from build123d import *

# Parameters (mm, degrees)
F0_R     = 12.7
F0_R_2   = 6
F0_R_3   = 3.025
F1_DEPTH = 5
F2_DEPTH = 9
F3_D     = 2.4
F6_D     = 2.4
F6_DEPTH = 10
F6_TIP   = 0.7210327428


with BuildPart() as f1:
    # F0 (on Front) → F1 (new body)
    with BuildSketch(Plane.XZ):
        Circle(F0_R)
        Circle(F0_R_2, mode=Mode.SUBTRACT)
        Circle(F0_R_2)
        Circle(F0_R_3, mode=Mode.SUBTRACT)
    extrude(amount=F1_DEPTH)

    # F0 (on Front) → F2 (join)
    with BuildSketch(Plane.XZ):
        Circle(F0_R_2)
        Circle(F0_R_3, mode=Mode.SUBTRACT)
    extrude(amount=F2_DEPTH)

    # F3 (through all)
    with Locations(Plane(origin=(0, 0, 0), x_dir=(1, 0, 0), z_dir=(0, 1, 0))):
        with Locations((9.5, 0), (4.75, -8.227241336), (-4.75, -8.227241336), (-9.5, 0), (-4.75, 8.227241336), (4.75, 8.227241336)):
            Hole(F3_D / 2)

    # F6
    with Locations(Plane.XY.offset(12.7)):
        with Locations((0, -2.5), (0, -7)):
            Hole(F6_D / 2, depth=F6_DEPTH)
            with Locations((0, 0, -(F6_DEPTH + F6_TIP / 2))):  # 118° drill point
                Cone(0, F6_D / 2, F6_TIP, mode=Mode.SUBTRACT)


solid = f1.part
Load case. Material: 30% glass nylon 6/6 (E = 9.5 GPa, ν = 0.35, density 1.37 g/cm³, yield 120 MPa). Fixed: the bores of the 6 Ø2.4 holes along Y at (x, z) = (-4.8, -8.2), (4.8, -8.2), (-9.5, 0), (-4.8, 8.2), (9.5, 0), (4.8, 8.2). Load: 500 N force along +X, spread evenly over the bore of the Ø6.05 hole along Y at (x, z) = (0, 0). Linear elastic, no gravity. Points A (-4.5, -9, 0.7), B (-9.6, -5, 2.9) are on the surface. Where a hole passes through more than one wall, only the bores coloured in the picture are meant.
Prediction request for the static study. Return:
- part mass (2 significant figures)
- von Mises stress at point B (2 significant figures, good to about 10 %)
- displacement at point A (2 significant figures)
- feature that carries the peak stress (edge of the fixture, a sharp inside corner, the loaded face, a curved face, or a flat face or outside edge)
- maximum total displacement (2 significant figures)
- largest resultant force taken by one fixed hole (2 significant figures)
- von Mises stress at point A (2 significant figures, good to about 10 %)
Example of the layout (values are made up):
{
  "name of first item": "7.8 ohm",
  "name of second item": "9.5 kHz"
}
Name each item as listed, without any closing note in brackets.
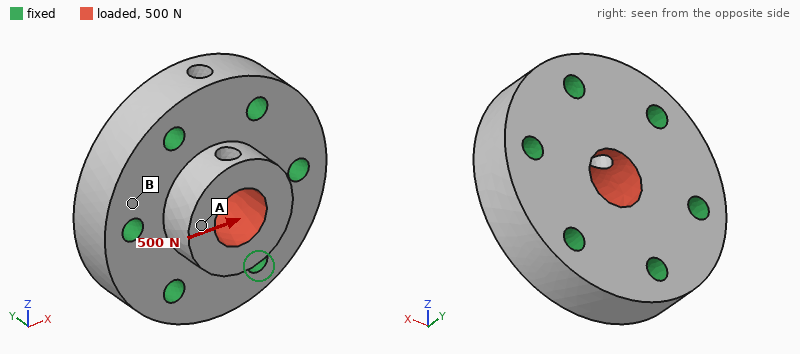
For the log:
{
  "part mass": "3.5 g",
  "von Mises stress at point B": "1.8 MPa",
  "displacement at point A": "7.9 µm",
  "feature that carries the peak stress": "the loaded face",
  "maximum total displacement": "8.6 µm",
  "largest resultant force taken by one fixed hole": "140 N",
  "von Mises stress at point A": "4.9 MPa"
}
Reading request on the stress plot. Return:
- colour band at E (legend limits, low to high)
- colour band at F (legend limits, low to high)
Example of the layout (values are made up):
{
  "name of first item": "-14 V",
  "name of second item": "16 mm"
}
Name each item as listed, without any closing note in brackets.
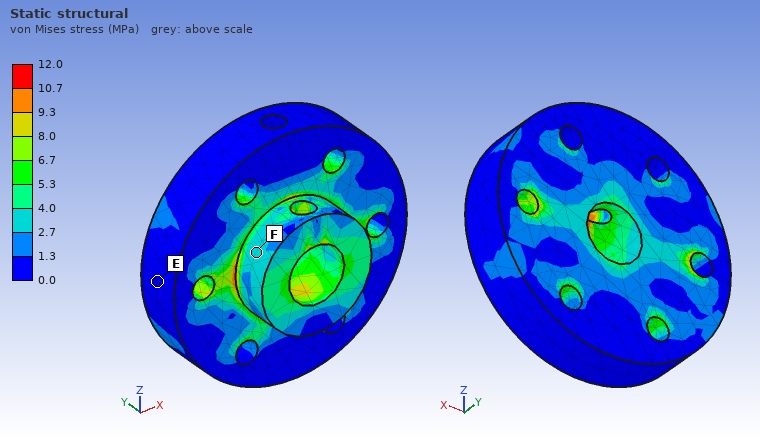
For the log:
{
  "colour band at E": "0.0 to 1.3 MPa",
  "colour band at F": "2.7 to 4.0 MPa"
}
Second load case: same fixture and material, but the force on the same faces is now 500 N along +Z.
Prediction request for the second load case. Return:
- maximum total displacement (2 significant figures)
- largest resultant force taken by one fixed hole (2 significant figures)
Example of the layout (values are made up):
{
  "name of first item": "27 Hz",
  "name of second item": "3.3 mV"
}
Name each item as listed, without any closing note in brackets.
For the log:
{
  "maximum total displacement": "8.2 µm",
  "largest resultant force taken by one fixed hole": "120 N"
}
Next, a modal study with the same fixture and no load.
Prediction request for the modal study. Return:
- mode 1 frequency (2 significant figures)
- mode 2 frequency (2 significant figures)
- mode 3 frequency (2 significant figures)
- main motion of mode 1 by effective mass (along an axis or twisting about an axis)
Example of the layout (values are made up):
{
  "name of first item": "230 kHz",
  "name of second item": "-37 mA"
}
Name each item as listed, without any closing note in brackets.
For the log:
{
  "mode 1 frequency": "45 kHz",
  "mode 2 frequency": "49 kHz",
  "mode 3 frequency": "50 kHz",
  "main motion of mode 1 by effective mass": "along Y"
}
